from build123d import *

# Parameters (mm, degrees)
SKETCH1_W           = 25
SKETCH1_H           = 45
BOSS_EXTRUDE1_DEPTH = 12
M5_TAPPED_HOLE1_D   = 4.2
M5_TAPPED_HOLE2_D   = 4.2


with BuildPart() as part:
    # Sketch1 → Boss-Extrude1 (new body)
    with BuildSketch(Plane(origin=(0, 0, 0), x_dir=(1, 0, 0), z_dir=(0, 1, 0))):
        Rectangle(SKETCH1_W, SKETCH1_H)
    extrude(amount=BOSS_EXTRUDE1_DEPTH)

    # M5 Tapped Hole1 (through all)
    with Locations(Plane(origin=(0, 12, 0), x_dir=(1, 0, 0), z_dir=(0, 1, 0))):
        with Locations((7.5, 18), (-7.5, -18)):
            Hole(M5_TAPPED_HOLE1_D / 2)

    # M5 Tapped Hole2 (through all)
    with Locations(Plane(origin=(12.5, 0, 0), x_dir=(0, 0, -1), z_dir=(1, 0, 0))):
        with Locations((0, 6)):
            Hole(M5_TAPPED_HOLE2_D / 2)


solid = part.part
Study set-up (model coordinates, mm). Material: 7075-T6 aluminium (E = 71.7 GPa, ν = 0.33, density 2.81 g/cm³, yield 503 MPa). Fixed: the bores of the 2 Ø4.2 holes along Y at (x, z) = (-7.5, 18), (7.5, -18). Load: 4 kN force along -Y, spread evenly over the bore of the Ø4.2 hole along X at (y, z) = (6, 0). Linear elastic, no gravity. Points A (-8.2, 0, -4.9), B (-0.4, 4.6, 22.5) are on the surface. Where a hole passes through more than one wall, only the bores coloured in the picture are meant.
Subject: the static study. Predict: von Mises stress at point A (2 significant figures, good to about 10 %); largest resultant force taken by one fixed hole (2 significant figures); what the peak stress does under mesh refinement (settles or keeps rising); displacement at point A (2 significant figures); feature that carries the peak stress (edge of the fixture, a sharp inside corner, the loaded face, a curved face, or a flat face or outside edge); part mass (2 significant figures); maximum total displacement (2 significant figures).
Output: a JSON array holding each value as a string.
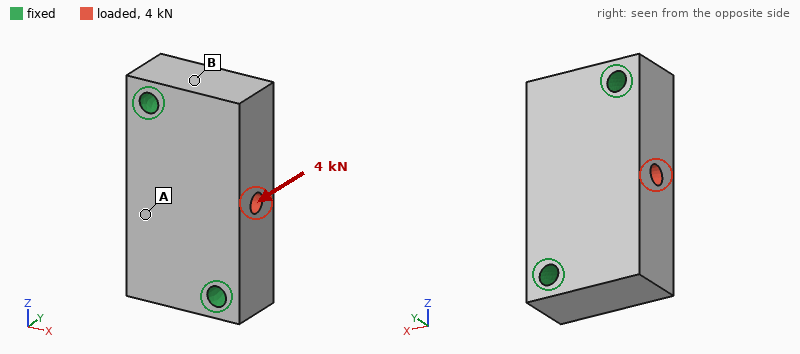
["26 MPa", "2.0 kN", "keeps rising", "13 µm", "edge of the fixture", "36 g", "15 µm"]
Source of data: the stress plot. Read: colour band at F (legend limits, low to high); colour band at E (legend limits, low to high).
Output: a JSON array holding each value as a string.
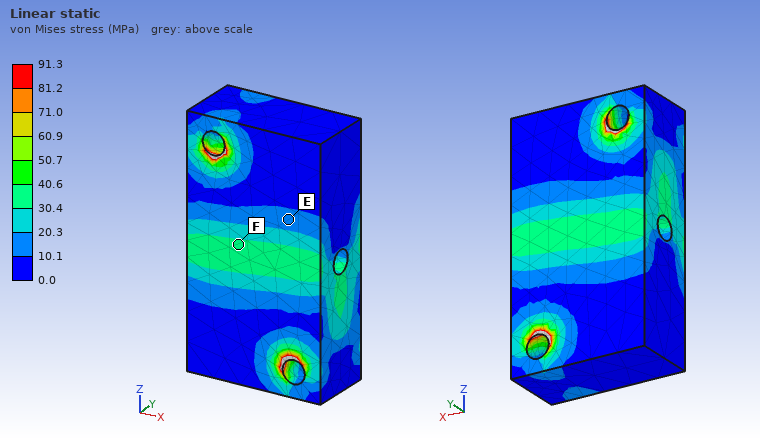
["30.4 to 40.6 MPa", "10.1 to 20.3 MPa"]
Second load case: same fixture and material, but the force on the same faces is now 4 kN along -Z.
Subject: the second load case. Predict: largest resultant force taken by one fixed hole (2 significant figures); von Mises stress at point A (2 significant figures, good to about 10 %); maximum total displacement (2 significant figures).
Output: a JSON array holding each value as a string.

["2.0 kN", "5.6 MPa", "5.1 µm"]
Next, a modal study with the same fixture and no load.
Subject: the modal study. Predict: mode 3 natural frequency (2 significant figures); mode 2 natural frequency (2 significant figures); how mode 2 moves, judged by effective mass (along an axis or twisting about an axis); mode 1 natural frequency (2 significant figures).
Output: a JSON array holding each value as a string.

["25 kHz", "20 kHz", "along Y", "18 kHz"]
